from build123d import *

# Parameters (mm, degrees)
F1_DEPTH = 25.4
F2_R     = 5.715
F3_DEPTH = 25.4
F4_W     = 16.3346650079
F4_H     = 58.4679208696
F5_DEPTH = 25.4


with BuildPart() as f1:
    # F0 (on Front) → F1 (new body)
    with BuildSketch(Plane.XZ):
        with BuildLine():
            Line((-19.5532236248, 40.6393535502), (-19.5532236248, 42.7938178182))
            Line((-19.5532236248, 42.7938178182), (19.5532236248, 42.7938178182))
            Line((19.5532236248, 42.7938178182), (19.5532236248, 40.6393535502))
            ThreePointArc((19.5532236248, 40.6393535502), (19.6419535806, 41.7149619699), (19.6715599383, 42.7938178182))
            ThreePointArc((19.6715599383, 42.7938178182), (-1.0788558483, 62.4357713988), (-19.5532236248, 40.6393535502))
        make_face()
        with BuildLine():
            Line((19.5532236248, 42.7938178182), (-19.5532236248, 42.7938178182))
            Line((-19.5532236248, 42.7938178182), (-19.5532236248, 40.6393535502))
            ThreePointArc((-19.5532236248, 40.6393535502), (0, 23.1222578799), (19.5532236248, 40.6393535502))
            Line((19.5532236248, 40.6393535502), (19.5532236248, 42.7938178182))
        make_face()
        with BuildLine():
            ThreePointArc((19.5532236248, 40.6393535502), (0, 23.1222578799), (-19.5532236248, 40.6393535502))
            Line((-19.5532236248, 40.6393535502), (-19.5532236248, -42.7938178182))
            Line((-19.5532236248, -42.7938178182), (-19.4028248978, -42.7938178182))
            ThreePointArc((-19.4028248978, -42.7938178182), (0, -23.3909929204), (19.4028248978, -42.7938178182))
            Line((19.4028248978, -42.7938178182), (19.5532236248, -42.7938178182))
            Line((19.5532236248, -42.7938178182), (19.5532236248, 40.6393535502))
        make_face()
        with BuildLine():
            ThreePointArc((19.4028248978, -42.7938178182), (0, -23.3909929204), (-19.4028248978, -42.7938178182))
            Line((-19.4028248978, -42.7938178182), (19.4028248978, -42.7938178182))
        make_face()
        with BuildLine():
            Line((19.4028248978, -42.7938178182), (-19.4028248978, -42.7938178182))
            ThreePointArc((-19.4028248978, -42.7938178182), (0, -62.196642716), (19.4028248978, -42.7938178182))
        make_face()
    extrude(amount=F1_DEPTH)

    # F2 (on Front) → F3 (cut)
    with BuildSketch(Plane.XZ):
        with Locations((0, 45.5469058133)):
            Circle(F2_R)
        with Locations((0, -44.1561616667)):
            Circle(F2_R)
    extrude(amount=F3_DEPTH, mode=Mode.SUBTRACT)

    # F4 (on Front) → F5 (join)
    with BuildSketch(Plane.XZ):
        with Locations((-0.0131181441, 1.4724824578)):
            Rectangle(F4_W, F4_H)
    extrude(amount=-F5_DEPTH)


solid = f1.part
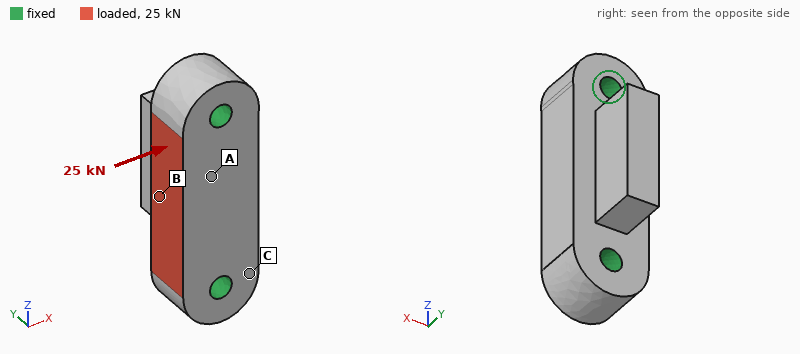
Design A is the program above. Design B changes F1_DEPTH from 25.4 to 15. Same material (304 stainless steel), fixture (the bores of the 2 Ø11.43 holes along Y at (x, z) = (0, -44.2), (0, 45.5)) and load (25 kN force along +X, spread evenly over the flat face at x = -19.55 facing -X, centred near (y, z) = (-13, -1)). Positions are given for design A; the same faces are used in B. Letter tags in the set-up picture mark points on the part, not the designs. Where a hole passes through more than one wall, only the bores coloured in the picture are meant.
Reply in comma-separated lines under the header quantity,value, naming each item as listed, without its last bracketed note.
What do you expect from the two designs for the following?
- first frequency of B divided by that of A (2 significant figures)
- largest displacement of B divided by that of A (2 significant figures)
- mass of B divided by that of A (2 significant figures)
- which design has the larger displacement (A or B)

quantity,value
first frequency of B divided by that of A,0.80
largest displacement of B divided by that of A,1.7
mass of B divided by that of A,0.66
which design has the larger displacement,B
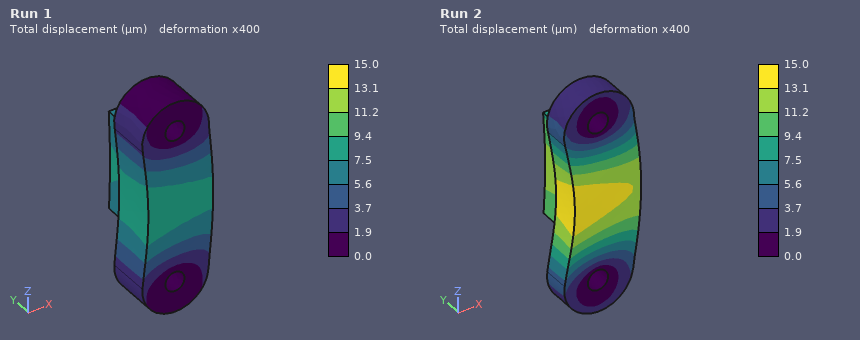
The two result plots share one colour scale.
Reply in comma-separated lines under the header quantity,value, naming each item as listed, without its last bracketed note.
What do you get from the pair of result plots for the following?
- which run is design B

quantity,value
which run is design B,Run 2
